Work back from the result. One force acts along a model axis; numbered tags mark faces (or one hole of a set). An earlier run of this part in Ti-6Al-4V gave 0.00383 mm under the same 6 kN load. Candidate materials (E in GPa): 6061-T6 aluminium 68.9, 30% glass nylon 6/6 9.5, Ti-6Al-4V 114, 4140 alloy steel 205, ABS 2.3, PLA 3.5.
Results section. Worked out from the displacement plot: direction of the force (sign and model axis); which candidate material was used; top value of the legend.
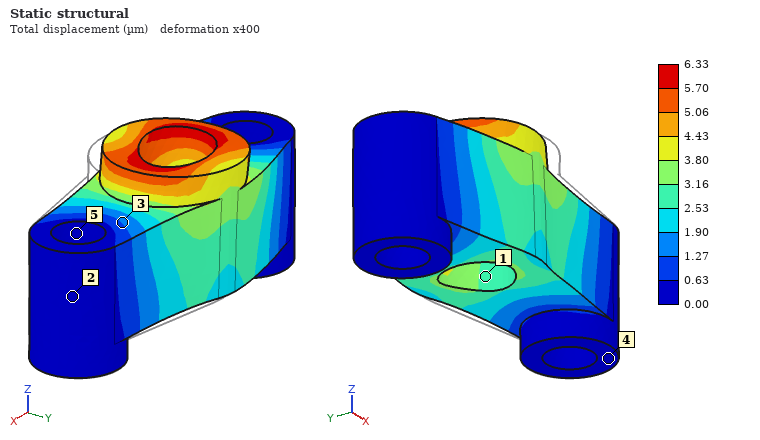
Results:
-X
6061-T6 aluminium
6.33 µm
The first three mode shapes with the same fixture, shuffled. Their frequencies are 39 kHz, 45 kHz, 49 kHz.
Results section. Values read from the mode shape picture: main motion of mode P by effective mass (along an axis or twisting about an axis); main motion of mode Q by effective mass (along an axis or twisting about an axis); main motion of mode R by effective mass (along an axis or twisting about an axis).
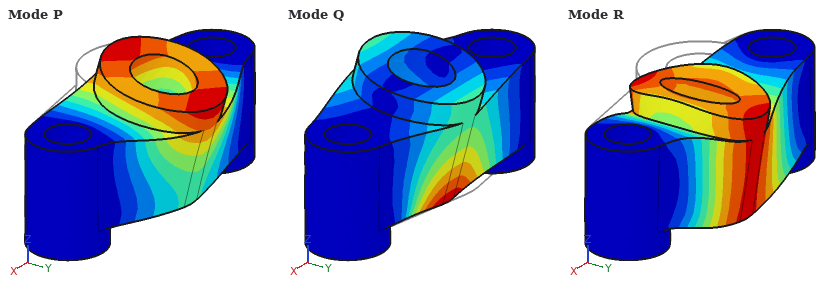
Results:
along Y
along Y
along Z
